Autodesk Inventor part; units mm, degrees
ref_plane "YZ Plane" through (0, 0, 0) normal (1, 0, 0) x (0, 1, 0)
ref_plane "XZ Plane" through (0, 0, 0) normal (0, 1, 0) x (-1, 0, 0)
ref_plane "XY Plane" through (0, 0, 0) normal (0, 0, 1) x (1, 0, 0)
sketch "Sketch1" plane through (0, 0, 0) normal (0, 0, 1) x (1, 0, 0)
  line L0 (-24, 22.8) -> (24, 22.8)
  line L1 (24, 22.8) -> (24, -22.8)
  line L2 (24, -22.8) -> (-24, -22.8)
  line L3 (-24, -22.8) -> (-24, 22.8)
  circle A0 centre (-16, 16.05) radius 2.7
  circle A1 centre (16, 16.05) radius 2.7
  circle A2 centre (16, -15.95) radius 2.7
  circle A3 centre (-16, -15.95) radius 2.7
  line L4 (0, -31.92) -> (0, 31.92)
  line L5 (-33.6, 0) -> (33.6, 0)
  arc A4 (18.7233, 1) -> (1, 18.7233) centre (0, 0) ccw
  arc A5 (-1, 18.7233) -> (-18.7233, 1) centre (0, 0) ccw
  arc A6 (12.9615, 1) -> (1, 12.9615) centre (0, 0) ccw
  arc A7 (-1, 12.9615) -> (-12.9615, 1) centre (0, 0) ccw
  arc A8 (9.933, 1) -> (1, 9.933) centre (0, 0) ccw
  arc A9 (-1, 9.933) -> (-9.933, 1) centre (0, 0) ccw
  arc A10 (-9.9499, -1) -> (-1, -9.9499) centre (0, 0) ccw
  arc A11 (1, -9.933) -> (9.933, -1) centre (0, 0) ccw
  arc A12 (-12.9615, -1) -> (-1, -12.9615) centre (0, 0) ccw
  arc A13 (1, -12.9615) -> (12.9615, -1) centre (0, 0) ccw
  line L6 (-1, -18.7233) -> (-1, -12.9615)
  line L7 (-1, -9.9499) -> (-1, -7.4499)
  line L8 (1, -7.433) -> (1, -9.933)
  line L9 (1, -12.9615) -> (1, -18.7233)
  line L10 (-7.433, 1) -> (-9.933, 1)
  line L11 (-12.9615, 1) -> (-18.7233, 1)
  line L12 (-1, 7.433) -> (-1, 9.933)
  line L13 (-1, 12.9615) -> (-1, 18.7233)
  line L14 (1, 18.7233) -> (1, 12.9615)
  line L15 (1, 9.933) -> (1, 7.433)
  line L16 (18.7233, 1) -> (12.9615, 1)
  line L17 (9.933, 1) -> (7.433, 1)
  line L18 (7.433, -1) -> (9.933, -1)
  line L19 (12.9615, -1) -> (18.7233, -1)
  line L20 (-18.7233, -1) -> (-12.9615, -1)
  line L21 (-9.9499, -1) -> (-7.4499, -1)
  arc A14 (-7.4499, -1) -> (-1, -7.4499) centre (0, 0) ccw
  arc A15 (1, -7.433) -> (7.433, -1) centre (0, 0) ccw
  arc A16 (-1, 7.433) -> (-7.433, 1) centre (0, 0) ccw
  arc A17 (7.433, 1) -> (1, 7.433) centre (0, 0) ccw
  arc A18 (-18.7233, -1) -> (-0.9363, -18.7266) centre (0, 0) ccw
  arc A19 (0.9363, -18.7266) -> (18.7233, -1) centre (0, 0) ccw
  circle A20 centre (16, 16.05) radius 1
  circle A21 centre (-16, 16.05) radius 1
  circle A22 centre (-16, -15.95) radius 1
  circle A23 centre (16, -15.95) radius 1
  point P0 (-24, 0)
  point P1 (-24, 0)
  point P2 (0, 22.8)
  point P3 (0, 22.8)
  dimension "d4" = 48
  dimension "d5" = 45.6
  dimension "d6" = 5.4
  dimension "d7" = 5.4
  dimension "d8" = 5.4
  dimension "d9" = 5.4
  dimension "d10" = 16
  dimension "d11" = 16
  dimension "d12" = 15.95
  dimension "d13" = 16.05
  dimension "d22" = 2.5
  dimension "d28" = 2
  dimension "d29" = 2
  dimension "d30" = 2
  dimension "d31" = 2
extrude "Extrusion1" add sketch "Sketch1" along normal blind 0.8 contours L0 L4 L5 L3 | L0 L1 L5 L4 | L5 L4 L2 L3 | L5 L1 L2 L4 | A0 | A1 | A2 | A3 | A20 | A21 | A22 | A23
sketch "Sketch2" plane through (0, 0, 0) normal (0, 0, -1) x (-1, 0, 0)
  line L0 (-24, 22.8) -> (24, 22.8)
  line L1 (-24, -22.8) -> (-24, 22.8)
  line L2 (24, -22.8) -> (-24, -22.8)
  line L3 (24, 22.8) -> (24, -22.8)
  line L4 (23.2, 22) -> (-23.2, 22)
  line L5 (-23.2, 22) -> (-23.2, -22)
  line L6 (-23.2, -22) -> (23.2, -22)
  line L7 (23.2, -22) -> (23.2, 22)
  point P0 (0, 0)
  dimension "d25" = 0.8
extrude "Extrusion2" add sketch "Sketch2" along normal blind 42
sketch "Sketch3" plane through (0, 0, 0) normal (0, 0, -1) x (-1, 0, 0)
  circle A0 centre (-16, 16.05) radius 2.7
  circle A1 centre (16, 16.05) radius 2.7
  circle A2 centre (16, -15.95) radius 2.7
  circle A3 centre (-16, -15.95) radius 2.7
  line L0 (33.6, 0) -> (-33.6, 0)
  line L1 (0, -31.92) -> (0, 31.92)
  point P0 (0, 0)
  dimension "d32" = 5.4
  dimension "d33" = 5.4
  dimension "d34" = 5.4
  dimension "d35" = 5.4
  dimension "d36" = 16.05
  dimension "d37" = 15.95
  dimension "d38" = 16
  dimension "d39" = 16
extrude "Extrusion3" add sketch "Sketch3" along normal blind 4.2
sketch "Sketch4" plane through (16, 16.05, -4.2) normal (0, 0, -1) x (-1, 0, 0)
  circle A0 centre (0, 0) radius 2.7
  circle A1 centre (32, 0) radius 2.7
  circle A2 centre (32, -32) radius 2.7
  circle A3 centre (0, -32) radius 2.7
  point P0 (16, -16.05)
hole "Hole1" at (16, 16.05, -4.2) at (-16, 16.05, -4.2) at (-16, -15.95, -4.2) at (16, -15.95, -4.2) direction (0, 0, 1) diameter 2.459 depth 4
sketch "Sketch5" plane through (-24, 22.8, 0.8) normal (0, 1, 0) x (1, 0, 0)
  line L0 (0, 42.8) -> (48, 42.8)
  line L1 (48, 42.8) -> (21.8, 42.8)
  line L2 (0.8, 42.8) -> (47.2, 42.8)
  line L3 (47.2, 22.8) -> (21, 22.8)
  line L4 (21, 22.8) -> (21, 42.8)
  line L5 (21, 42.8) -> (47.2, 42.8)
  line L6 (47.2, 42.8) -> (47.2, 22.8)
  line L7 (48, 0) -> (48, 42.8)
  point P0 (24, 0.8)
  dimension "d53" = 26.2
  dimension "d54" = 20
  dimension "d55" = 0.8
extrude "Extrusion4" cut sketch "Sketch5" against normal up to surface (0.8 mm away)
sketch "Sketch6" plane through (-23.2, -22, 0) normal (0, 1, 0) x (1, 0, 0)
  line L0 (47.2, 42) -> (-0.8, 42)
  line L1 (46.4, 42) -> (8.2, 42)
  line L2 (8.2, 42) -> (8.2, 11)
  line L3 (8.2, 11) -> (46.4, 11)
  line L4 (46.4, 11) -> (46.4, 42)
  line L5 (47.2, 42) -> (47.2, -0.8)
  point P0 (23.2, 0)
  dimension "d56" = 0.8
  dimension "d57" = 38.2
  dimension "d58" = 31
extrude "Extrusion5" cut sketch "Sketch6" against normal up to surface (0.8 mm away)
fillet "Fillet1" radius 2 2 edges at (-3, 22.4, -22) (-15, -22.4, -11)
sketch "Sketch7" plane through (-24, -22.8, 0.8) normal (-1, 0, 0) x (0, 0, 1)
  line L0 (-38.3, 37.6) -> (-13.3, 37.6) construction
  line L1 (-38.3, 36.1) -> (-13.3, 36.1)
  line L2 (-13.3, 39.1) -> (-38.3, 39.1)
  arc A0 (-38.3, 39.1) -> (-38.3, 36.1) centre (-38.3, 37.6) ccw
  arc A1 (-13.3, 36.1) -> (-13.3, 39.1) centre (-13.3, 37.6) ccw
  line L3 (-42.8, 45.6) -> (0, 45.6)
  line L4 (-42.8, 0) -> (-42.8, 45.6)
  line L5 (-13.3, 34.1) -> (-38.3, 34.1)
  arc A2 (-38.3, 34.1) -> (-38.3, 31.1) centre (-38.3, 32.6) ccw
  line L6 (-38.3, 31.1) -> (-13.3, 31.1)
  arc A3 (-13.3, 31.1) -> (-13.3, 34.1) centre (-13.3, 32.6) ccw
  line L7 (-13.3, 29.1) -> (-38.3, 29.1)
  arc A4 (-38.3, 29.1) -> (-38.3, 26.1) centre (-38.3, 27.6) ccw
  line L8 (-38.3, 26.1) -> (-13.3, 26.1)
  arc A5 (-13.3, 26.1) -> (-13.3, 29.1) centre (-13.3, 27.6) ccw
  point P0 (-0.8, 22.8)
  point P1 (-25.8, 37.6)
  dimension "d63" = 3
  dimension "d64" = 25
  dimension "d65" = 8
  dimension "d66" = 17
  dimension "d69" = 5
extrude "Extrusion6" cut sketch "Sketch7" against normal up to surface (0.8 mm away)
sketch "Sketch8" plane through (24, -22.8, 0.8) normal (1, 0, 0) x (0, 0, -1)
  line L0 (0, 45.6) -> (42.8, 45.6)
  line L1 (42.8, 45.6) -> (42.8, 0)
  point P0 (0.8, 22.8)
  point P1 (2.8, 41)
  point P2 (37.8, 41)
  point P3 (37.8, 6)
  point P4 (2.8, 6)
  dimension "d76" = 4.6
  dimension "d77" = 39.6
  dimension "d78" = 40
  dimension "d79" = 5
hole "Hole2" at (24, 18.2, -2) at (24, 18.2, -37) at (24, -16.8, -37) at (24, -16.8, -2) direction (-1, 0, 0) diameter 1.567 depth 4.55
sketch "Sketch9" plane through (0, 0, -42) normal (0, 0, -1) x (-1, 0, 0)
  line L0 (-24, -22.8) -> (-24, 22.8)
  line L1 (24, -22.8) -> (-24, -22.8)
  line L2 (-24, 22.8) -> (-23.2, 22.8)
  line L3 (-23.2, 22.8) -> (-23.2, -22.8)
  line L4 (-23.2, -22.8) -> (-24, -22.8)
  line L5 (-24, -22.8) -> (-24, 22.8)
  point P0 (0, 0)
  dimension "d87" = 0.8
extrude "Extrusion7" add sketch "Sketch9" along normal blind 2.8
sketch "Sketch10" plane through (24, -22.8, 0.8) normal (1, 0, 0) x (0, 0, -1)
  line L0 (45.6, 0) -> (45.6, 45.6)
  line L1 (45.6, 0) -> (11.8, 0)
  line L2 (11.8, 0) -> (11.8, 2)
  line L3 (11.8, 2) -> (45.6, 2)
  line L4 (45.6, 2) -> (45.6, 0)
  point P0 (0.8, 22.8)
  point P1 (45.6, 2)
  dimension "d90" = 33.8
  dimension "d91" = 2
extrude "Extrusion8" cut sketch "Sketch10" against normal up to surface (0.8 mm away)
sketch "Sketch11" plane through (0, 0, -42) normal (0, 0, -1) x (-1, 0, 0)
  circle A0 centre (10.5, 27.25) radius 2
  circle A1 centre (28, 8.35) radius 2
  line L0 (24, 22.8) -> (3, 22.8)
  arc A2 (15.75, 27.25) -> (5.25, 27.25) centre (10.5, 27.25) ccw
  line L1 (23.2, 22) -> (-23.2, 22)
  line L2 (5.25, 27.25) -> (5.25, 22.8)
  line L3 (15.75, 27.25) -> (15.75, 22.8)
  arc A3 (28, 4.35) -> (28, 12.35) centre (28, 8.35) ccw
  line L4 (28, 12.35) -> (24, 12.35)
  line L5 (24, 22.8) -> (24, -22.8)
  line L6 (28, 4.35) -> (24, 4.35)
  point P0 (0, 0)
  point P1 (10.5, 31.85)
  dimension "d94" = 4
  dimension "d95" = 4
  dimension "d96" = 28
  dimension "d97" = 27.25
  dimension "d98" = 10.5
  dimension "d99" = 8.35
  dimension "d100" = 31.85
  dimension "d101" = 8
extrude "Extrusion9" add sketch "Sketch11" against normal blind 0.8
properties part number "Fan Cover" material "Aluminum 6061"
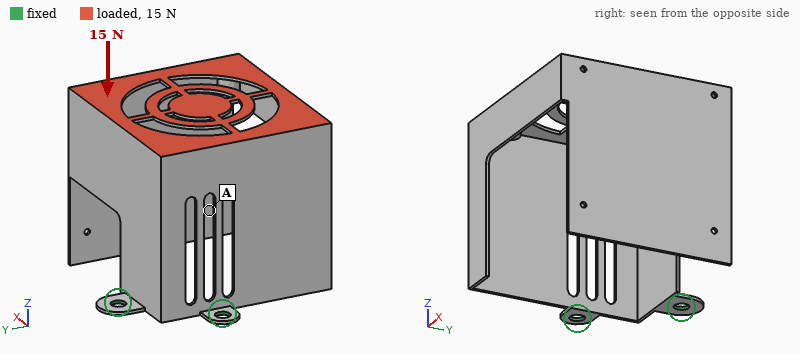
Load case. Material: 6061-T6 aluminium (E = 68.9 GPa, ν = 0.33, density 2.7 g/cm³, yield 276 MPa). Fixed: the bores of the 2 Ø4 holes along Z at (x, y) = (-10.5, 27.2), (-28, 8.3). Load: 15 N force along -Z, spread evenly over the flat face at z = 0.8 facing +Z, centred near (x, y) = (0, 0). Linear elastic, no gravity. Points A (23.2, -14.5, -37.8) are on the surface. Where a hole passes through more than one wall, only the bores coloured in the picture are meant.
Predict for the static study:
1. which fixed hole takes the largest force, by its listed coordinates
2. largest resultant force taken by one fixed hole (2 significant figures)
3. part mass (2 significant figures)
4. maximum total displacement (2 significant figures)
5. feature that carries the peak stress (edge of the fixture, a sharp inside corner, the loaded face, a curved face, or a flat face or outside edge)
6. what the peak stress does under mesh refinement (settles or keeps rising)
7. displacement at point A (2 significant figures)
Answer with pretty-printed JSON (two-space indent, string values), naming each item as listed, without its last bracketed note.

{
  "which fixed hole takes the largest force, by its listed coordinates": "(-28, 8.3)",
  "largest resultant force taken by one fixed hole": "9.4 N",
  "part mass": "17 g",
  "maximum total displacement": "1.0 mm",
  "feature that carries the peak stress": "edge of the fixture",
  "what the peak stress does under mesh refinement": "keeps rising",
  "displacement at point A": "0.84 mm"
}
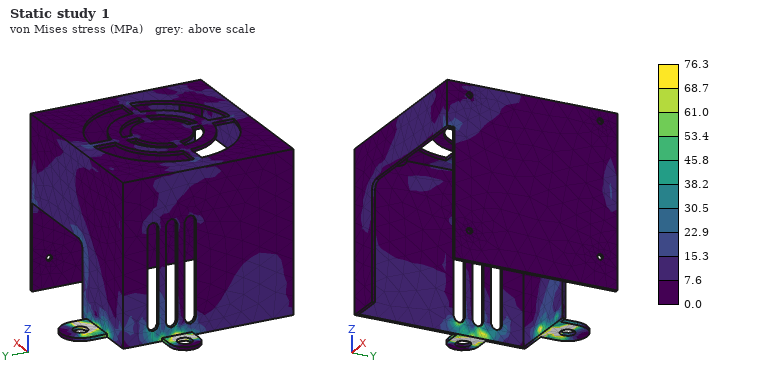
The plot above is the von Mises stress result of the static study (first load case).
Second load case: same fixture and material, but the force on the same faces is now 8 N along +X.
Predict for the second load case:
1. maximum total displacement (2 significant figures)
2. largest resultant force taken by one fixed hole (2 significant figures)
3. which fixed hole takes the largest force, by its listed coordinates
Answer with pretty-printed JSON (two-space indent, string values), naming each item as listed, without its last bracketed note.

{
  "maximum total displacement": "1.0 mm",
  "largest resultant force taken by one fixed hole": "11 N",
  "which fixed hole takes the largest force, by its listed coordinates": "(-28, 8.3)"
}
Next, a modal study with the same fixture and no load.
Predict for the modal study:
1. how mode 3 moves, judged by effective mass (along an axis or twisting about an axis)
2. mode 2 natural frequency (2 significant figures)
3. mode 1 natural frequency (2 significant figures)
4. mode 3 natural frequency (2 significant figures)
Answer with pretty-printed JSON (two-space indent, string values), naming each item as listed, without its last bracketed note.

{
  "how mode 3 moves, judged by effective mass": "along X",
  "mode 2 natural frequency": "170 Hz",
  "mode 1 natural frequency": "110 Hz",
  "mode 3 natural frequency": "320 Hz"
}
